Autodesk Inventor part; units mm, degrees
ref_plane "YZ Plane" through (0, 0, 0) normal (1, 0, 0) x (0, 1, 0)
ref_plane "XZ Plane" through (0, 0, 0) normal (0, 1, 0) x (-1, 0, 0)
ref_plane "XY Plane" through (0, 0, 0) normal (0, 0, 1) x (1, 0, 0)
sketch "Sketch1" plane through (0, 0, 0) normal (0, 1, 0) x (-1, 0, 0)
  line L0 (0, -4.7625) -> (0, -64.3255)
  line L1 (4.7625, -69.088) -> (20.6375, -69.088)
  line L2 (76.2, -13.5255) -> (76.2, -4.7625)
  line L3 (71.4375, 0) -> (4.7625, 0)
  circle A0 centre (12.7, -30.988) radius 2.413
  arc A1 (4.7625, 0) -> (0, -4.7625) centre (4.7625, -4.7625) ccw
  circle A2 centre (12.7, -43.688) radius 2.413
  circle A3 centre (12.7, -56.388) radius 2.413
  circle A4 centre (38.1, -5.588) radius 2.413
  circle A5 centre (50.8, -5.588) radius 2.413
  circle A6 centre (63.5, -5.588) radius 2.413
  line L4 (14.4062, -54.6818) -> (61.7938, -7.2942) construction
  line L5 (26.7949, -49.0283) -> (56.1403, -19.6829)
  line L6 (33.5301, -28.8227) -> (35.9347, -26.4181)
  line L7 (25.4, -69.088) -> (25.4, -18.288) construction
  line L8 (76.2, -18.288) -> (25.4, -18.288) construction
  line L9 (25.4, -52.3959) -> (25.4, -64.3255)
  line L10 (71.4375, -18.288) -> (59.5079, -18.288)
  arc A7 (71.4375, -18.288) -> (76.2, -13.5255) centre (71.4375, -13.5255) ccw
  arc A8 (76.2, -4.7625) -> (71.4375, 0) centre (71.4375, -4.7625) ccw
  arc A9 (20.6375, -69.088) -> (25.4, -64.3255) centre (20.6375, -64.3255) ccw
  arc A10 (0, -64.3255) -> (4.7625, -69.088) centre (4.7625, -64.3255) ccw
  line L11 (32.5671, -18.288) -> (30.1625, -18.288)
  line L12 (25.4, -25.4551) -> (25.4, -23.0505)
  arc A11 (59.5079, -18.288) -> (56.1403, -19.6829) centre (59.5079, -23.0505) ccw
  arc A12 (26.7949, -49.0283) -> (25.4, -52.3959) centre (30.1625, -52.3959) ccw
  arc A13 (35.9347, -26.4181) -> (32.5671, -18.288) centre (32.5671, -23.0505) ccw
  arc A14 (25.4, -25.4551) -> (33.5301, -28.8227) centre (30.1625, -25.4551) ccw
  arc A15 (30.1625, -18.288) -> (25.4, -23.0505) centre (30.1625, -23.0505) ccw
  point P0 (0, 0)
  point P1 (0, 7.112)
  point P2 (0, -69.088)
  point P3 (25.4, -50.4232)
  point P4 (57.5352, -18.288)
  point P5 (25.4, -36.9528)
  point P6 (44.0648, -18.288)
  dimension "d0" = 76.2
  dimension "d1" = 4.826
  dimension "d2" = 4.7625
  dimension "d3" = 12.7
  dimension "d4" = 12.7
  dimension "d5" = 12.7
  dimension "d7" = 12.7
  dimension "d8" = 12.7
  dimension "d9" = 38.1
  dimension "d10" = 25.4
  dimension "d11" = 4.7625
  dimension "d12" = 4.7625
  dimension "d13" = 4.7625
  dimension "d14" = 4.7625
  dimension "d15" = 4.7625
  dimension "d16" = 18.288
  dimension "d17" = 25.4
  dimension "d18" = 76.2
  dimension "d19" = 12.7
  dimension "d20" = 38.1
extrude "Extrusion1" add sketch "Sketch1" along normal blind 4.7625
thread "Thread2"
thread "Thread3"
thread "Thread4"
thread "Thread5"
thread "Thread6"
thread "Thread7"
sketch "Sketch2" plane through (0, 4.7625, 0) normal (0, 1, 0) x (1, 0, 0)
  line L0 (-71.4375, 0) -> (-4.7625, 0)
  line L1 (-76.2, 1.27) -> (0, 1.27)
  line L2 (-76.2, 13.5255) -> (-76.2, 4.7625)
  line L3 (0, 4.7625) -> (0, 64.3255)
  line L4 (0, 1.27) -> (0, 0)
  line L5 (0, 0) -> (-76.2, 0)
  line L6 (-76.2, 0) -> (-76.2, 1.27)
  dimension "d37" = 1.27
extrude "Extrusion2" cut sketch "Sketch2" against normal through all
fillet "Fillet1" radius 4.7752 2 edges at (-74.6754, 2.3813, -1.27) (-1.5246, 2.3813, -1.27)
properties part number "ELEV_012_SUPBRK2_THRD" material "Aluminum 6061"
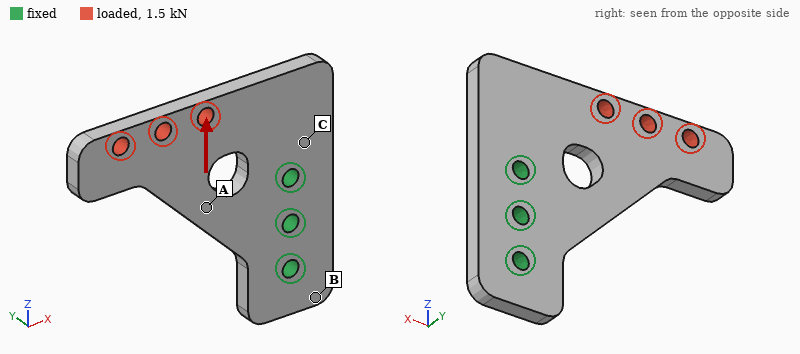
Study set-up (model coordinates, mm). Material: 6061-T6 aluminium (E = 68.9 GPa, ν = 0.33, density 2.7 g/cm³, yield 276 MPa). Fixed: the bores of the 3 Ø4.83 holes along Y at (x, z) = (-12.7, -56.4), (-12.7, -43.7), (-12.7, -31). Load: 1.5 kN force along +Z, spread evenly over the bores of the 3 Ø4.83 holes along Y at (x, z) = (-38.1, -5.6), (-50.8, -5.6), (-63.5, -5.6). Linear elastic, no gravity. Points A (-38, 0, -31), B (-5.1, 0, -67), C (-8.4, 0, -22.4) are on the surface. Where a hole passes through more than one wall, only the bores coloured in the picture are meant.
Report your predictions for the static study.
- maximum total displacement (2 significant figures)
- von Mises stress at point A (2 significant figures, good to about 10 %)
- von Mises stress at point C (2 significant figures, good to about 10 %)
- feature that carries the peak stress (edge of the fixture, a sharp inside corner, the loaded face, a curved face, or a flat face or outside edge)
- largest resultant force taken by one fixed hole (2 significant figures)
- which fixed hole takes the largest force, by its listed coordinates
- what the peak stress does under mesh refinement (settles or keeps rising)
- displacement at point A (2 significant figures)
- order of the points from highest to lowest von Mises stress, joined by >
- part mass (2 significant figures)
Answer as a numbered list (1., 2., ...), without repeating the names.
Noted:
1. 0.12 mm
2. 38 MPa
3. 21 MPa
4. edge of the fixture
5. 2.4 kN
6. (-12.7, -31)
7. keeps rising
8. 0.031 mm
9. A > C > B
10. 37 g
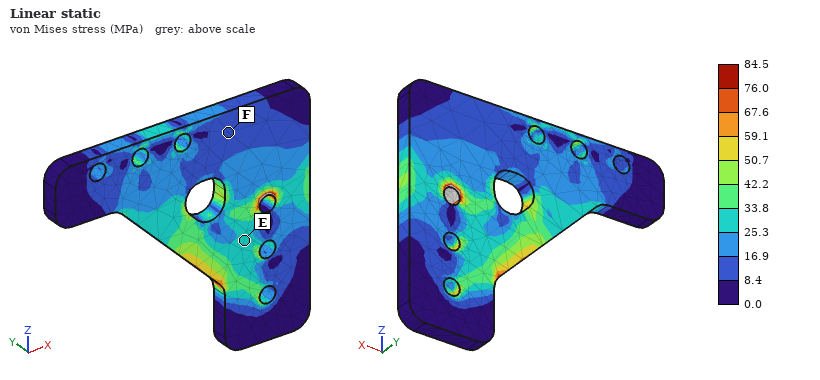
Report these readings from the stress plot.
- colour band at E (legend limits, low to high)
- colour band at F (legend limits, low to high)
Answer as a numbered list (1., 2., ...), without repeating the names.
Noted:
1. 25.3 to 33.8 MPa
2. 8.4 to 16.9 MPa
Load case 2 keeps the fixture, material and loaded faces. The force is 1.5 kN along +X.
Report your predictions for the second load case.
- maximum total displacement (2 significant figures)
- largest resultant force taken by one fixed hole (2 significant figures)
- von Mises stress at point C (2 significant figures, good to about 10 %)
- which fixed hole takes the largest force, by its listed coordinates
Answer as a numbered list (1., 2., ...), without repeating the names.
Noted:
1. 0.10 mm
2. 2.9 kN
3. 26 MPa
4. (-12.7, -31)
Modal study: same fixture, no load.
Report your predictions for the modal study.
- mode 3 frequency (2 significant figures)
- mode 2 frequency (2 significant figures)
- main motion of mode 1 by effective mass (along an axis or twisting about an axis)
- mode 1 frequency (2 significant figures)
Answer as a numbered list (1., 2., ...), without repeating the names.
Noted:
1. 5500 Hz
2. 3700 Hz
3. along Y
4. 1100 Hz
